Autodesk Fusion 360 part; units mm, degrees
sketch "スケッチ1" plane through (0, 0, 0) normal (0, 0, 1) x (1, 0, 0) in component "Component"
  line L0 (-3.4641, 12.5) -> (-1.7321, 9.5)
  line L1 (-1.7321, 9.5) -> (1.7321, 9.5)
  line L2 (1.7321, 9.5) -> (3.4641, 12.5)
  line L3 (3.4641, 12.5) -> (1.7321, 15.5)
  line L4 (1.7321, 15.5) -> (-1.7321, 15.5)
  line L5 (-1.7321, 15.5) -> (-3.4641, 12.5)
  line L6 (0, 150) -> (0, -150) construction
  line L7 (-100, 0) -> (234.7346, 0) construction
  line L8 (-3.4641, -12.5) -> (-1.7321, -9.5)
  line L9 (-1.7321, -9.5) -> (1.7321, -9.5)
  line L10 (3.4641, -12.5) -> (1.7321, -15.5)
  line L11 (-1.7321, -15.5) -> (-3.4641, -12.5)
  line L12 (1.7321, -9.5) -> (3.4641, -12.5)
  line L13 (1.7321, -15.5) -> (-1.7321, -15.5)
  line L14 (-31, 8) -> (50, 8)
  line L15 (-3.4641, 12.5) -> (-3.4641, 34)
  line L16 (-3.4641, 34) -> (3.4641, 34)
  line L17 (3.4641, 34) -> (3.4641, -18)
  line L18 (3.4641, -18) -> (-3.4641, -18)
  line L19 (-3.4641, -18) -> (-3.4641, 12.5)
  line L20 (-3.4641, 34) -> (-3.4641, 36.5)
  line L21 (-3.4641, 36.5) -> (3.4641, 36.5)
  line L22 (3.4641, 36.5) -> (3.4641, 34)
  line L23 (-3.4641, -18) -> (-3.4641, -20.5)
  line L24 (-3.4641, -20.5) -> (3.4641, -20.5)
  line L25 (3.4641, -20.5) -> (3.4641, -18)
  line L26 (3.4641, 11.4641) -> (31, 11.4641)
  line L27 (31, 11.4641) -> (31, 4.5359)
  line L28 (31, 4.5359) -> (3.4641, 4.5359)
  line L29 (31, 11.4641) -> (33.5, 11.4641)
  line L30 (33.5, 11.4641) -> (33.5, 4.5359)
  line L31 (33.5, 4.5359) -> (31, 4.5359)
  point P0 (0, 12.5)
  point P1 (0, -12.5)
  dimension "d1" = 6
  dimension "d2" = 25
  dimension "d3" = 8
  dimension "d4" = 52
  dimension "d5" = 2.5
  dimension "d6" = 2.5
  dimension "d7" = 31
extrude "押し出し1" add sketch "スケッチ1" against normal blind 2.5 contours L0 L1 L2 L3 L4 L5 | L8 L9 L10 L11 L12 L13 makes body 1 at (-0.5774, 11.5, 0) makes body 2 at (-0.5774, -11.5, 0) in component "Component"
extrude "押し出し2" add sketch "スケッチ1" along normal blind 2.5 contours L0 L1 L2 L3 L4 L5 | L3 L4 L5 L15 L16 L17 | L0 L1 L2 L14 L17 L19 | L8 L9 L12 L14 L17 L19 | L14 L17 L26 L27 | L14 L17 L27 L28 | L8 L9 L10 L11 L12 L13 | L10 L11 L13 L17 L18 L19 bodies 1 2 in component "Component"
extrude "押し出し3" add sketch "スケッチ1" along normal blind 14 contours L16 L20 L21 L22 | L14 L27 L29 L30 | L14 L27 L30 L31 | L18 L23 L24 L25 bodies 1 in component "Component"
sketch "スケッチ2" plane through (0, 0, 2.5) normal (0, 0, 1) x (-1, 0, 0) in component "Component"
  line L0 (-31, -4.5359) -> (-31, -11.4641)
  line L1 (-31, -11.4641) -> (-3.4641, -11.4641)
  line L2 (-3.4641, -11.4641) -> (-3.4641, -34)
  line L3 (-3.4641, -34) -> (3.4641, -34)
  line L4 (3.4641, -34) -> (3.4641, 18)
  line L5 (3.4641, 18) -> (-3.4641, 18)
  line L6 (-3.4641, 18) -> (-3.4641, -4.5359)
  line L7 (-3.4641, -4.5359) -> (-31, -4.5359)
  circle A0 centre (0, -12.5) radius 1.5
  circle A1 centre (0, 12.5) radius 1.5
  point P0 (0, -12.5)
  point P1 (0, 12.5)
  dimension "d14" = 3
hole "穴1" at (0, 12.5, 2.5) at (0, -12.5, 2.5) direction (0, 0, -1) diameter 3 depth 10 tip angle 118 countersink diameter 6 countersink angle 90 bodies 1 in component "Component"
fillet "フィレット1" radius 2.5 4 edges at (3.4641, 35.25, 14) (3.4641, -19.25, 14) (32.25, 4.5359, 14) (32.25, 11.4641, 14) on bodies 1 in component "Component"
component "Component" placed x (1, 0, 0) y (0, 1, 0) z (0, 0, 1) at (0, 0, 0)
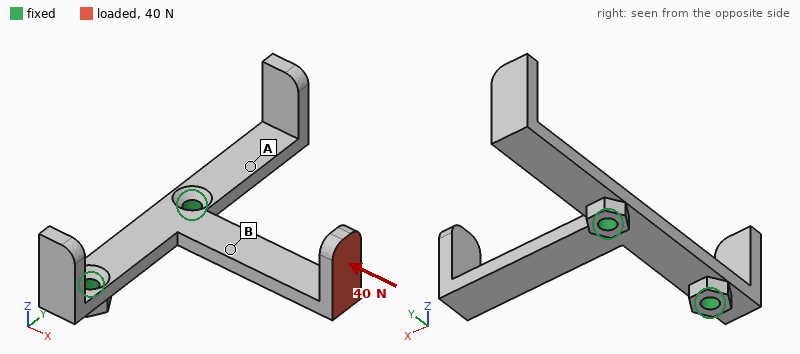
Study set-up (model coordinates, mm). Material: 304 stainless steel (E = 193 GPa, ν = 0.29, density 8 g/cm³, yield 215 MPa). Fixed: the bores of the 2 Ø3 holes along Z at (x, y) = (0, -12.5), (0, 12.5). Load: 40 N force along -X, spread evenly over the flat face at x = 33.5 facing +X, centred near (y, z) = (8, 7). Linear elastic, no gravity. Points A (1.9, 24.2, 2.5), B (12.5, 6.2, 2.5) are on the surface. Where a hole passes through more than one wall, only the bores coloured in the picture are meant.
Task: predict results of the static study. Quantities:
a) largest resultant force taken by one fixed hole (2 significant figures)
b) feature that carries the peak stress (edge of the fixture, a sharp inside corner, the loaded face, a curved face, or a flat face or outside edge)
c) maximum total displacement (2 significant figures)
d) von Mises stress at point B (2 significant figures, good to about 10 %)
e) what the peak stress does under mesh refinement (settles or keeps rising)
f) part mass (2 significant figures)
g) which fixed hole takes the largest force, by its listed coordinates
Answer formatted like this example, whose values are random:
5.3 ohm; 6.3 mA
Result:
35 N; edge of the fixture; 93 µm; 33 MPa; keeps rising; 17 g; (0, 12.5)
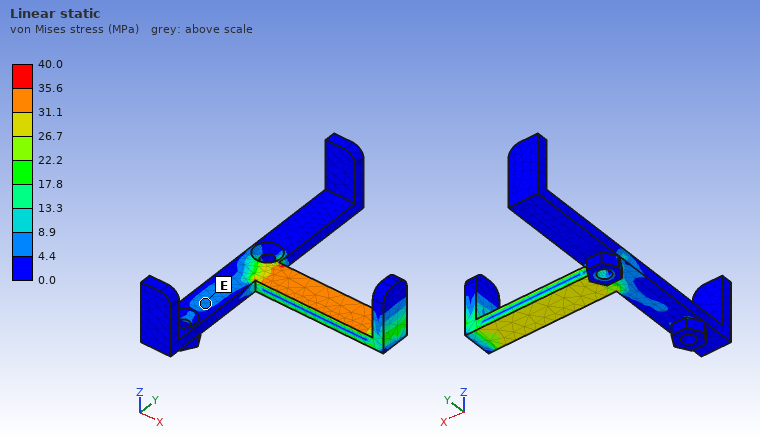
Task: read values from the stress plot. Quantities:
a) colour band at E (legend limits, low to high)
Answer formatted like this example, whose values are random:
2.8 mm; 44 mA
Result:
4.4 to 8.9 MPa
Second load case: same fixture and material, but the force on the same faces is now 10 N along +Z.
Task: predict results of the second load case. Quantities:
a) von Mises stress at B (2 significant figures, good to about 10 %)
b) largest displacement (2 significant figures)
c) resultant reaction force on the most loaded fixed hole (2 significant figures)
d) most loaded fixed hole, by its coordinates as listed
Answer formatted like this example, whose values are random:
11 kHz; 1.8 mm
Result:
29 MPa; 84 µm; 11 N; (0, 12.5)
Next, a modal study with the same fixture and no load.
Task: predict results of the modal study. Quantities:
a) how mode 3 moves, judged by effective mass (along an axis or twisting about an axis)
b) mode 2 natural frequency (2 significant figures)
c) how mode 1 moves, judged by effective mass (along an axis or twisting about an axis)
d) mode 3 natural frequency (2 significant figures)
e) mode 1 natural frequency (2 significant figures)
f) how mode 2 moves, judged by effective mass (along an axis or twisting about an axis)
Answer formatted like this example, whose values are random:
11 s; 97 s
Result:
along Y; 2000 Hz; along Z; 2800 Hz; 1100 Hz; along Z
